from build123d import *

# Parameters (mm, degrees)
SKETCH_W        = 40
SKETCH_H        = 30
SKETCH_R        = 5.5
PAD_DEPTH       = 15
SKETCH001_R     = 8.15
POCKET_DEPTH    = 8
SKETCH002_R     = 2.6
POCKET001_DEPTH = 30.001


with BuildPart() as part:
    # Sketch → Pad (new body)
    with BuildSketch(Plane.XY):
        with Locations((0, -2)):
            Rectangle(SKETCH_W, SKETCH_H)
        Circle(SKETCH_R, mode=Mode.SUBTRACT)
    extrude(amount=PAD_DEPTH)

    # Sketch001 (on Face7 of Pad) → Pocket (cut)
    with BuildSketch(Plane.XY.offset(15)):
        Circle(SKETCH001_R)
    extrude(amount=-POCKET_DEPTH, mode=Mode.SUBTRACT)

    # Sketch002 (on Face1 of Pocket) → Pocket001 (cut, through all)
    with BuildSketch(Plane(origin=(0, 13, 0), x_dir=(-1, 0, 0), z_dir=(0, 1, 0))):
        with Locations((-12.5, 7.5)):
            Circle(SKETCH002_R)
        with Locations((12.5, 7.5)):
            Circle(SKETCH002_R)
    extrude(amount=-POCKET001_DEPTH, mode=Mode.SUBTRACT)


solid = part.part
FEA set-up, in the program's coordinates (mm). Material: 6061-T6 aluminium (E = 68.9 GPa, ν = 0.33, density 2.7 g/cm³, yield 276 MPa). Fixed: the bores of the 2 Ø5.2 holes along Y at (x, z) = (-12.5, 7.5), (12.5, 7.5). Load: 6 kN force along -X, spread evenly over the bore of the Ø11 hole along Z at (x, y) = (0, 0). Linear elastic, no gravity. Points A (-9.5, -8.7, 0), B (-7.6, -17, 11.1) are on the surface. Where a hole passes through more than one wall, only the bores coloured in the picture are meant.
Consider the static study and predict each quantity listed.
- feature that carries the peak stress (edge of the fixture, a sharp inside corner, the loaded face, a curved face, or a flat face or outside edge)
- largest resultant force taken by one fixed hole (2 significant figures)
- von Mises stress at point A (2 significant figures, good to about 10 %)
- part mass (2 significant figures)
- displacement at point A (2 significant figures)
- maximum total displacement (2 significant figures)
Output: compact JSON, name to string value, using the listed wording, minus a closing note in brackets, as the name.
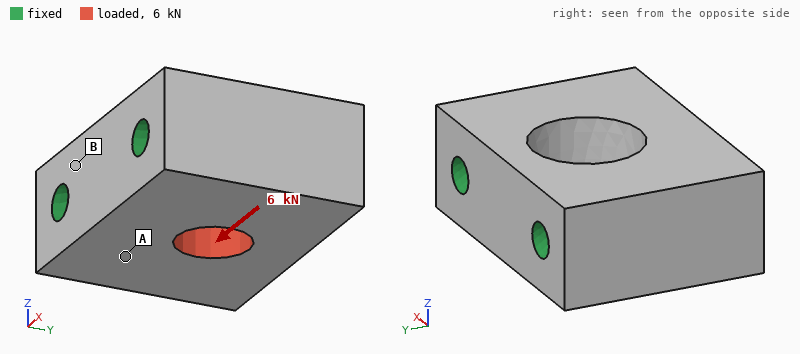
{"feature that carries the peak stress": "the loaded face", "largest resultant force taken by one fixed hole": "3.0 kN", "von Mises stress at point A": "11 MPa", "part mass": "39 g", "displacement at point A": "1.3 µm", "maximum total displacement": "4.1 µm"}
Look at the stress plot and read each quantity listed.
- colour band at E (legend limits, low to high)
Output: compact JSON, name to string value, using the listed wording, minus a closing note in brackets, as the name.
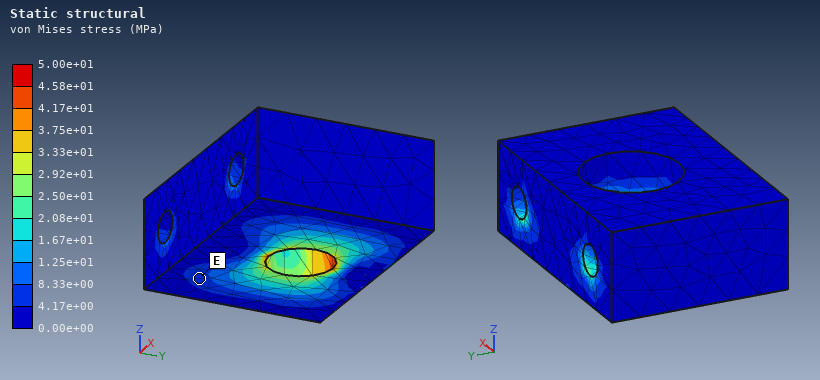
{"colour band at E": "4.17e+00 to 8.33e+00 MPa"}
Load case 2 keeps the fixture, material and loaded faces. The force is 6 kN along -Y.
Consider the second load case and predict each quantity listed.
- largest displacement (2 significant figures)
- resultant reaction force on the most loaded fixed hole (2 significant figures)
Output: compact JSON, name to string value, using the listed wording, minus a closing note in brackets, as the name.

{"largest displacement": "7.8 µm", "resultant reaction force on the most loaded fixed hole": "3.0 kN"}
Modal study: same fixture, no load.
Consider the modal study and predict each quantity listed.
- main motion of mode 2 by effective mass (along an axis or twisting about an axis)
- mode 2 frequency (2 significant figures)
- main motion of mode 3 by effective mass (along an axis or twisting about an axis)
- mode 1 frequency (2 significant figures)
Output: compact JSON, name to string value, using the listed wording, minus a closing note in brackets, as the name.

{"main motion of mode 2 by effective mass": "twisting about X", "mode 2 frequency": "57 kHz", "main motion of mode 3 by effective mass": "along Y", "mode 1 frequency": "53 kHz"}
